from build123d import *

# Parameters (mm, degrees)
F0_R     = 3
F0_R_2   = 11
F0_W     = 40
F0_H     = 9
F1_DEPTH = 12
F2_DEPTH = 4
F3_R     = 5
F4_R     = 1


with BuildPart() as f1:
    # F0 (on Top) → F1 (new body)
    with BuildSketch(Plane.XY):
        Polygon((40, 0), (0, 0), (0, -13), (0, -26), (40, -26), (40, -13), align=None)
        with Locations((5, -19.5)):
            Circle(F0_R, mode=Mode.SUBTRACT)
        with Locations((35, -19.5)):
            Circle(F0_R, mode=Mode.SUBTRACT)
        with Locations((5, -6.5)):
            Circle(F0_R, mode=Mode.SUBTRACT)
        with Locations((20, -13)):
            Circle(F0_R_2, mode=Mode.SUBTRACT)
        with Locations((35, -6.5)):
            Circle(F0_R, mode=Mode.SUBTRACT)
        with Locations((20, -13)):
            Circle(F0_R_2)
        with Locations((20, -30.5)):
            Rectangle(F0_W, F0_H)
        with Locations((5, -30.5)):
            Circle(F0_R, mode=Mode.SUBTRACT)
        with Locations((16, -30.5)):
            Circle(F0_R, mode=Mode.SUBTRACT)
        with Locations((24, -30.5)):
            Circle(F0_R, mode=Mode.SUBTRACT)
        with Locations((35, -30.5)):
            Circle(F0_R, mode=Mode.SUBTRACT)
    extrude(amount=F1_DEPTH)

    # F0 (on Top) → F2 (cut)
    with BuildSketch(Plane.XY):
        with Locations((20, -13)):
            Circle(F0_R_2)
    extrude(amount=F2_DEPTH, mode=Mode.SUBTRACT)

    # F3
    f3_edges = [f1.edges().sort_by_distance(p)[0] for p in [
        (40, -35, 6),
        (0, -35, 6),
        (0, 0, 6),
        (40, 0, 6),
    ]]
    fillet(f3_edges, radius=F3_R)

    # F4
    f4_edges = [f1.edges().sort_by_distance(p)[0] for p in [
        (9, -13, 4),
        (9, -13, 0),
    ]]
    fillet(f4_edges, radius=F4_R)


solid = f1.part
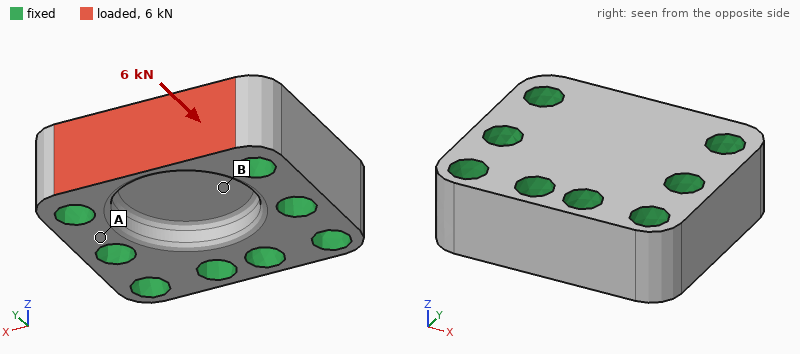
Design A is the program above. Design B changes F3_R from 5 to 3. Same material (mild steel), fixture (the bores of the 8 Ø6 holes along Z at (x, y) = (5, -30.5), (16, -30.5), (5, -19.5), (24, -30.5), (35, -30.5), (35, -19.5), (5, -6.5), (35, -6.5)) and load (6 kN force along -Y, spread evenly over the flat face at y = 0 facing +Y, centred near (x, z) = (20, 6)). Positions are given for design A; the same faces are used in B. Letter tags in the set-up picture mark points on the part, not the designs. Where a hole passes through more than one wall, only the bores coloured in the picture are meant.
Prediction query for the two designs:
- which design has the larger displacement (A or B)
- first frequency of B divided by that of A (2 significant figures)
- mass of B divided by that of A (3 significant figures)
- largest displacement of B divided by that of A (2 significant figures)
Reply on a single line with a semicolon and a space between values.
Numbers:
A; 1.0; 1.01; 0.88
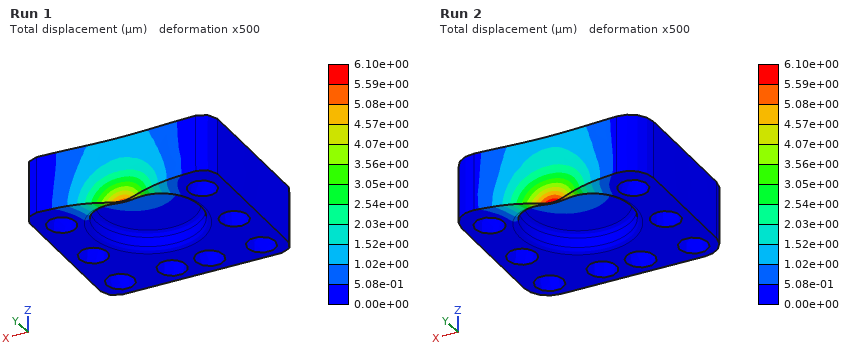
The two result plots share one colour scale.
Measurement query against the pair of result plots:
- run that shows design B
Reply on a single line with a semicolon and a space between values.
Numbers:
Run 1
